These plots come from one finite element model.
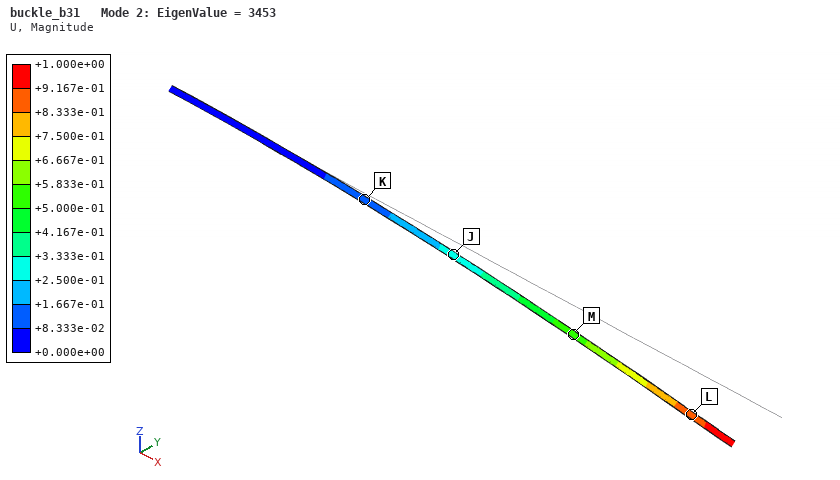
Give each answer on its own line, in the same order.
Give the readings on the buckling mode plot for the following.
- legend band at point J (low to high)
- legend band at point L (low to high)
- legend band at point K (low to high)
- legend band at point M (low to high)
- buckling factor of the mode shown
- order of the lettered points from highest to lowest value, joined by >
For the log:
+2.500e-01 to +3.333e-01
+8.333e-01 to +9.167e-01
+8.333e-02 to +1.667e-01
+5.000e-01 to +5.833e-01
3453
L > M > J > K
